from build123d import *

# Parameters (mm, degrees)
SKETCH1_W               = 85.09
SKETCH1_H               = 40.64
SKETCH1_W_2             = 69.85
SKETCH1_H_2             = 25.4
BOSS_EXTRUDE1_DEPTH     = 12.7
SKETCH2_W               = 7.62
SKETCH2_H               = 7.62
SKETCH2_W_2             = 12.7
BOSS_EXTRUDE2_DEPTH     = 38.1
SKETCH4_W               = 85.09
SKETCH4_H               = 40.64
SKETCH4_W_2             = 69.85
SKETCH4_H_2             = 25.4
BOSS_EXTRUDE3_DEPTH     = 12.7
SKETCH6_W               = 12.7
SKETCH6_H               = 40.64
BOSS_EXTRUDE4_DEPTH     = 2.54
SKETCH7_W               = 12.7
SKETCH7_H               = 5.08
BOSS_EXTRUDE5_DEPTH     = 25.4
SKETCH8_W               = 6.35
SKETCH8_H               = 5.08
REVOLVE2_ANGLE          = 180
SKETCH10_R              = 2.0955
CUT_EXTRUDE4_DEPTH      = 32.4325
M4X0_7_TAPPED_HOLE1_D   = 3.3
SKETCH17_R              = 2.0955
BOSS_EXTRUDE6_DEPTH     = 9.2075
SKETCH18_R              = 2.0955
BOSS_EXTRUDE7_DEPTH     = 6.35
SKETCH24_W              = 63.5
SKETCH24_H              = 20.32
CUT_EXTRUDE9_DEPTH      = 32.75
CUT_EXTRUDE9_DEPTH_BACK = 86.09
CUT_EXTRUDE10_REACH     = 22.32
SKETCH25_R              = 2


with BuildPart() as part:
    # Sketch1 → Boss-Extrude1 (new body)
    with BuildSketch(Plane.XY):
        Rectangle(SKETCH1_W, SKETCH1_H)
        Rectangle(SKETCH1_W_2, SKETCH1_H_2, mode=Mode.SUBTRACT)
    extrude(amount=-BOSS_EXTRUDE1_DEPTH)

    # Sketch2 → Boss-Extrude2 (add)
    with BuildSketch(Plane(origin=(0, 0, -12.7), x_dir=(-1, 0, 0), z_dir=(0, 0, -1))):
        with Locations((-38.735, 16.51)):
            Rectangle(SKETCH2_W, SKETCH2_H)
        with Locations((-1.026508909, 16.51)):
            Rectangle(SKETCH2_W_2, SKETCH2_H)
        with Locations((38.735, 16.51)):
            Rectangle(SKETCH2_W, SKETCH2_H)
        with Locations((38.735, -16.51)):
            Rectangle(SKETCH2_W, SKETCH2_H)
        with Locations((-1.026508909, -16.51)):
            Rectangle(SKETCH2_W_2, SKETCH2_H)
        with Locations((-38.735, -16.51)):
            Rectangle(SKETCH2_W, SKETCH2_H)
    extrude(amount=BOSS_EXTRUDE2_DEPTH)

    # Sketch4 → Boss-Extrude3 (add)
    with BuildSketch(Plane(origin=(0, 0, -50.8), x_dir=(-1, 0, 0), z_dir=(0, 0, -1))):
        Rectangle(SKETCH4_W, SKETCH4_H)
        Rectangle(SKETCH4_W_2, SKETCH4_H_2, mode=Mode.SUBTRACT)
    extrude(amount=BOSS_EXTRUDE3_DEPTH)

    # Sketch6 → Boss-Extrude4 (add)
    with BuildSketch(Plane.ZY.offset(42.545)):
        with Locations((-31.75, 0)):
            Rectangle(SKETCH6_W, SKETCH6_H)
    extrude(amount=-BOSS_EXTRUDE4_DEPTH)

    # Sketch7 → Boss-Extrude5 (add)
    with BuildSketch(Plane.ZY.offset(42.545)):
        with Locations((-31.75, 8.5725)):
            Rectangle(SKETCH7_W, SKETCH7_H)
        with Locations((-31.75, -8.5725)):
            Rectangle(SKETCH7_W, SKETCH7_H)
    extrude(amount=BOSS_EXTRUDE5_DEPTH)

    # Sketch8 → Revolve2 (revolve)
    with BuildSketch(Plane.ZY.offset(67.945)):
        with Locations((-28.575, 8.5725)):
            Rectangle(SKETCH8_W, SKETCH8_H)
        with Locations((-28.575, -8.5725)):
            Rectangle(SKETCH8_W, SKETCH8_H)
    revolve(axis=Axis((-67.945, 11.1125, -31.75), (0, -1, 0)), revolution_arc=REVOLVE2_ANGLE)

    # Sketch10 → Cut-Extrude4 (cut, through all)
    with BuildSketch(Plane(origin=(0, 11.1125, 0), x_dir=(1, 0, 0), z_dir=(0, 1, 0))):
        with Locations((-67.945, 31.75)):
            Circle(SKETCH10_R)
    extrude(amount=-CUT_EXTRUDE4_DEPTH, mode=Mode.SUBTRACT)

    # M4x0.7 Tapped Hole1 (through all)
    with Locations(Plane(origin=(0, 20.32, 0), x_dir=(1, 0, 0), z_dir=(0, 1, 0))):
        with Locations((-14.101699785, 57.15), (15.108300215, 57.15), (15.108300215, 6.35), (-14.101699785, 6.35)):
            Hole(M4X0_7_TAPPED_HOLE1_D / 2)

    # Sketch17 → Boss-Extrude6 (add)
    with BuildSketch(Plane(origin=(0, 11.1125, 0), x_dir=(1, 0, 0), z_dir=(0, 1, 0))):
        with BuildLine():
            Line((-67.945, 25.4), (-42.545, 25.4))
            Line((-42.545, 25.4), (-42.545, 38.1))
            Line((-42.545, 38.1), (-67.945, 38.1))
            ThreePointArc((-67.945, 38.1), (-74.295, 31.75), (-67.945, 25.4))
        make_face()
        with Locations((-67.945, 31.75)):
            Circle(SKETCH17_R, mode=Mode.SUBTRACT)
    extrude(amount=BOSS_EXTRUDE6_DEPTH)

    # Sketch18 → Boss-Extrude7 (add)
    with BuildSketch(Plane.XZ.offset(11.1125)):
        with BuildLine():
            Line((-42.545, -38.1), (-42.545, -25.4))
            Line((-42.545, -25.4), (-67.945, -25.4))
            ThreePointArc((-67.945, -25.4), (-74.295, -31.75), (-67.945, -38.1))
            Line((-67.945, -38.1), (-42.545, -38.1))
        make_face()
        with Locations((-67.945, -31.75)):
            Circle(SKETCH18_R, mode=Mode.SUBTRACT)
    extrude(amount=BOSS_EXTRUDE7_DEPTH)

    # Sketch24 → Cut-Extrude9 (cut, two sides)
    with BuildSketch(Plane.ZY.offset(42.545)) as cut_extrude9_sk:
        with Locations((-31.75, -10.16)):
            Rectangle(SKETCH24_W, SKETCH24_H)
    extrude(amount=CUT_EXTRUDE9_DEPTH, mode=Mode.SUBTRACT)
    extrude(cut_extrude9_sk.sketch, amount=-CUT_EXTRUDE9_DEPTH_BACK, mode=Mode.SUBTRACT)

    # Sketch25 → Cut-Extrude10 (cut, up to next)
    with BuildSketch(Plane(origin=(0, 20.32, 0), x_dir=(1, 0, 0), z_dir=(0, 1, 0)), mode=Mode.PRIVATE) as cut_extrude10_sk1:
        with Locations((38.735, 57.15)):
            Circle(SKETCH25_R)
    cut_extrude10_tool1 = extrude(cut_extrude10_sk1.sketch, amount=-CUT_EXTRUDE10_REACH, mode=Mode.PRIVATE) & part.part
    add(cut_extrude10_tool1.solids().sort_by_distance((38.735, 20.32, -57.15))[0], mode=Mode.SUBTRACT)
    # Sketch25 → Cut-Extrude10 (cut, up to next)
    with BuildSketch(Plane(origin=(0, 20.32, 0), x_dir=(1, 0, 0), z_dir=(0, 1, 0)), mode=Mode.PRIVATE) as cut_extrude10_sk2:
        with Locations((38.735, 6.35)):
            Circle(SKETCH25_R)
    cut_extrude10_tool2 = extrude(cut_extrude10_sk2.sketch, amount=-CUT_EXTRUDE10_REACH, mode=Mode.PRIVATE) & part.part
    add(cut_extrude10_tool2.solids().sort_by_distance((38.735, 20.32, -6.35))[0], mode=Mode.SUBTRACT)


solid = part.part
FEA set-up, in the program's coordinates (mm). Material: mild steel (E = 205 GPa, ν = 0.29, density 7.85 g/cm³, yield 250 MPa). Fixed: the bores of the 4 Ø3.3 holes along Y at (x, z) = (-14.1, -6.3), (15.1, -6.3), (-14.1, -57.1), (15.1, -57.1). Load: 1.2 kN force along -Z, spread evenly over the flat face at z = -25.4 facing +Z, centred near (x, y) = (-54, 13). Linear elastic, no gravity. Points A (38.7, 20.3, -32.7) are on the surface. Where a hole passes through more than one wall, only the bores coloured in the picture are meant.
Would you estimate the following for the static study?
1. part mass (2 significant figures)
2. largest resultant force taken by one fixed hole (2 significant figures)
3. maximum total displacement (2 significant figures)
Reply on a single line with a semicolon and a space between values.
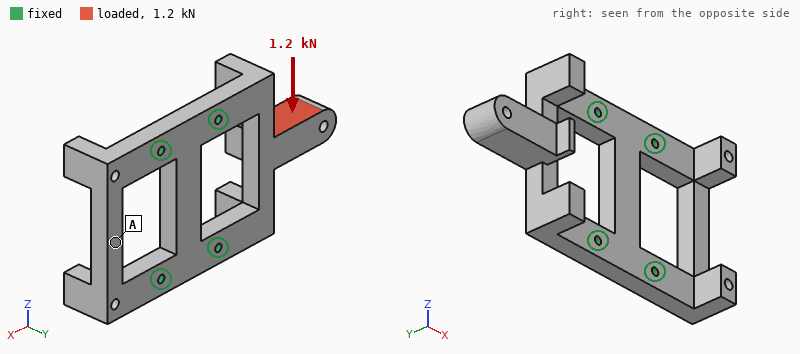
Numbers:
270 g; 990 N; 39 µm
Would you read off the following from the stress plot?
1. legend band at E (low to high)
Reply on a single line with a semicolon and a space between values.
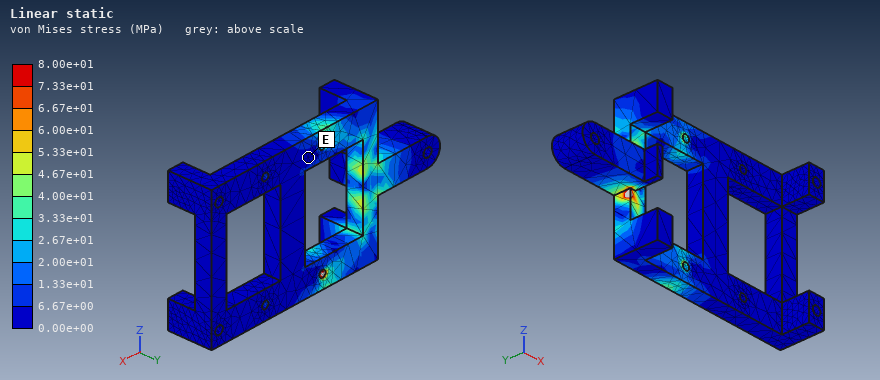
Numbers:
0.00e+00 to 6.67e+00 MPa
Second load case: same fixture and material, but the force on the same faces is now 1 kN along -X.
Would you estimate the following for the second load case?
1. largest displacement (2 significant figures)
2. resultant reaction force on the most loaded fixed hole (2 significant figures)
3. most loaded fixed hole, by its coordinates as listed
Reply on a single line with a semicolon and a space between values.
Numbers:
63 µm; 690 N; (-14.1, -6.3)
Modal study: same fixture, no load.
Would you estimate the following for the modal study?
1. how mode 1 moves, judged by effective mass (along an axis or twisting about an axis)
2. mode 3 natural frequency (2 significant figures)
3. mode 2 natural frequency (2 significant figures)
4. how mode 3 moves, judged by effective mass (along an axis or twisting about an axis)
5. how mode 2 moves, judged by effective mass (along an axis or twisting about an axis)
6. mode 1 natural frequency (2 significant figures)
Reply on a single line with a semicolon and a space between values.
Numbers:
along Y; 4500 Hz; 4100 Hz; along Z; along Y; 1400 Hz
